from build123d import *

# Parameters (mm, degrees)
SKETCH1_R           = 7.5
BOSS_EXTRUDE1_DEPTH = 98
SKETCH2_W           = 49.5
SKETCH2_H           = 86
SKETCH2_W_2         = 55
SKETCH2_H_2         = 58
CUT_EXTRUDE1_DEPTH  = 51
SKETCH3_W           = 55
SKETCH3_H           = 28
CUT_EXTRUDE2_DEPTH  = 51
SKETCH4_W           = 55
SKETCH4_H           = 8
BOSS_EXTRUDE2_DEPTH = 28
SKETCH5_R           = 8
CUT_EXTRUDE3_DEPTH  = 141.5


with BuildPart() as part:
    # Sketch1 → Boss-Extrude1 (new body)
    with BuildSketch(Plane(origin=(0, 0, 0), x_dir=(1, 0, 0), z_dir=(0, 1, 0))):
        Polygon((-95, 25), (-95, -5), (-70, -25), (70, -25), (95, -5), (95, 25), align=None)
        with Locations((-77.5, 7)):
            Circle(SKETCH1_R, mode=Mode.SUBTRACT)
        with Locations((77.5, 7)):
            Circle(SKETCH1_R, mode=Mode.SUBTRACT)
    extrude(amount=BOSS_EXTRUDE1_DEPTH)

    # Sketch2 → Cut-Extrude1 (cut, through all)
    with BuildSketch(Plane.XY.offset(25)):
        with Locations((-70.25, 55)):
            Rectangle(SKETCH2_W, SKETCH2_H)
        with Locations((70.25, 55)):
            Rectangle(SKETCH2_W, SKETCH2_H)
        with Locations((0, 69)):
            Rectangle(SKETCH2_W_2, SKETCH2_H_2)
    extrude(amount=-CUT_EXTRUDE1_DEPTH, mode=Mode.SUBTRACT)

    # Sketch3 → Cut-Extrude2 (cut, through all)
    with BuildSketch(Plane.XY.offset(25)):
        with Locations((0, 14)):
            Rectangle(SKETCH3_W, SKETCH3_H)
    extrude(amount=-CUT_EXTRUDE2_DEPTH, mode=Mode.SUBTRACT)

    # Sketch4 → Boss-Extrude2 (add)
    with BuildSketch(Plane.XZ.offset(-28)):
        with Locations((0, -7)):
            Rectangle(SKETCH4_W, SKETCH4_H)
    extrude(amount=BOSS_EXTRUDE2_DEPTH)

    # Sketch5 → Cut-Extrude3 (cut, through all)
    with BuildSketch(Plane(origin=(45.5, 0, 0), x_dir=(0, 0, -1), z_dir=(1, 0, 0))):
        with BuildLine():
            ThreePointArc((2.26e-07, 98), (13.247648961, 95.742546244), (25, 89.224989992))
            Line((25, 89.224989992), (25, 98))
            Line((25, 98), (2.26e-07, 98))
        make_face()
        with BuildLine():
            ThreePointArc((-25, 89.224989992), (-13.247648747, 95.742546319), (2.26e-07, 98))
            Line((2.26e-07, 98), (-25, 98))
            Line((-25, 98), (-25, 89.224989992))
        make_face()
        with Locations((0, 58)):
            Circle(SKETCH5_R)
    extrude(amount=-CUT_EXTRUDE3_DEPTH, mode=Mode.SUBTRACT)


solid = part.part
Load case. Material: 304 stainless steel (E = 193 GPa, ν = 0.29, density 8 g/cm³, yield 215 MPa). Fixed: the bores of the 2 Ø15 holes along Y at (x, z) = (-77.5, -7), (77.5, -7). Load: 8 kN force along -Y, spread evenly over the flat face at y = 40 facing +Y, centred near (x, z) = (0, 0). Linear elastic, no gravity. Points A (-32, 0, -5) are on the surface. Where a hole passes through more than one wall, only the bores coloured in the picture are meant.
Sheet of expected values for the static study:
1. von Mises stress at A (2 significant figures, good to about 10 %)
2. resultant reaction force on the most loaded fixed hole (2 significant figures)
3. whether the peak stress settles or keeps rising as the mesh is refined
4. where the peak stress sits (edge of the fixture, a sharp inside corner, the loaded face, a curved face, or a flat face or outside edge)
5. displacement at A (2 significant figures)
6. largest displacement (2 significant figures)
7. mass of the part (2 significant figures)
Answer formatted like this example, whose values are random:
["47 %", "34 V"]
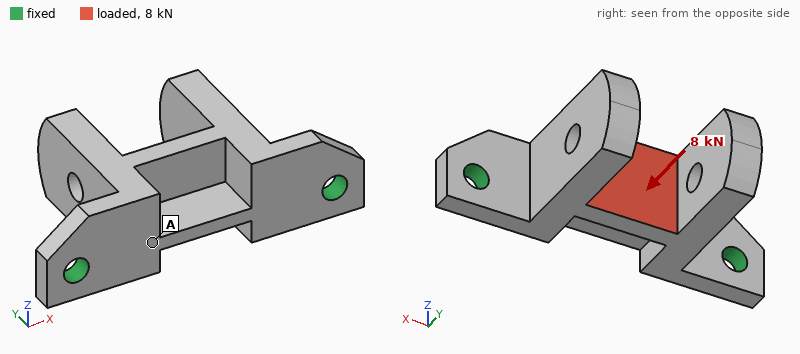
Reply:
["11 MPa", "5.9 kN", "keeps rising", "edge of the fixture", "18 µm", "36 µm", "2.1 kg"]
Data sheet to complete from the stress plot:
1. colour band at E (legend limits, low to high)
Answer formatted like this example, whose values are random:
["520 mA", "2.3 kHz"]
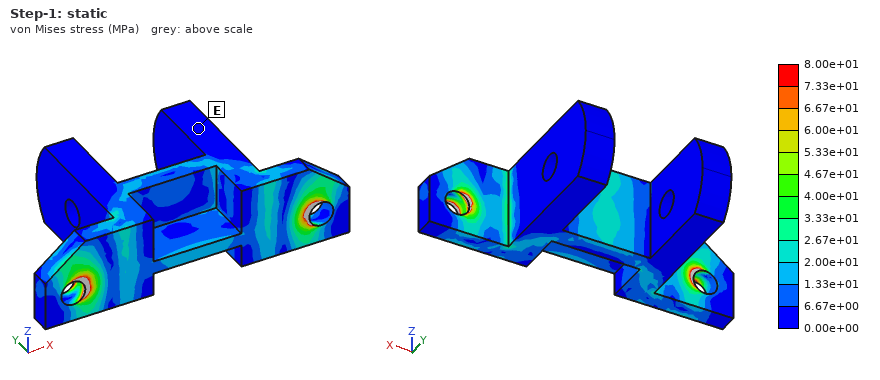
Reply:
["0.00e+00 to 6.67e+00 MPa"]
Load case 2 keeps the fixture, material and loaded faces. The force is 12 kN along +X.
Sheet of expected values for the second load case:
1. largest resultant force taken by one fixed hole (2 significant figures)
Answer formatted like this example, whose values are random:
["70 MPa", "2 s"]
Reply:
["6.9 kN"]
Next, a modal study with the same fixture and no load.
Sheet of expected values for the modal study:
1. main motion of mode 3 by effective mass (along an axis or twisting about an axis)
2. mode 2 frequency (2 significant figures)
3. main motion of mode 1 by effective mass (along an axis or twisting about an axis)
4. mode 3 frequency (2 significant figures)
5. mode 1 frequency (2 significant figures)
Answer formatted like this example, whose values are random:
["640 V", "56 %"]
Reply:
["along X", "1900 Hz", "along Z", "2100 Hz", "900 Hz"]
